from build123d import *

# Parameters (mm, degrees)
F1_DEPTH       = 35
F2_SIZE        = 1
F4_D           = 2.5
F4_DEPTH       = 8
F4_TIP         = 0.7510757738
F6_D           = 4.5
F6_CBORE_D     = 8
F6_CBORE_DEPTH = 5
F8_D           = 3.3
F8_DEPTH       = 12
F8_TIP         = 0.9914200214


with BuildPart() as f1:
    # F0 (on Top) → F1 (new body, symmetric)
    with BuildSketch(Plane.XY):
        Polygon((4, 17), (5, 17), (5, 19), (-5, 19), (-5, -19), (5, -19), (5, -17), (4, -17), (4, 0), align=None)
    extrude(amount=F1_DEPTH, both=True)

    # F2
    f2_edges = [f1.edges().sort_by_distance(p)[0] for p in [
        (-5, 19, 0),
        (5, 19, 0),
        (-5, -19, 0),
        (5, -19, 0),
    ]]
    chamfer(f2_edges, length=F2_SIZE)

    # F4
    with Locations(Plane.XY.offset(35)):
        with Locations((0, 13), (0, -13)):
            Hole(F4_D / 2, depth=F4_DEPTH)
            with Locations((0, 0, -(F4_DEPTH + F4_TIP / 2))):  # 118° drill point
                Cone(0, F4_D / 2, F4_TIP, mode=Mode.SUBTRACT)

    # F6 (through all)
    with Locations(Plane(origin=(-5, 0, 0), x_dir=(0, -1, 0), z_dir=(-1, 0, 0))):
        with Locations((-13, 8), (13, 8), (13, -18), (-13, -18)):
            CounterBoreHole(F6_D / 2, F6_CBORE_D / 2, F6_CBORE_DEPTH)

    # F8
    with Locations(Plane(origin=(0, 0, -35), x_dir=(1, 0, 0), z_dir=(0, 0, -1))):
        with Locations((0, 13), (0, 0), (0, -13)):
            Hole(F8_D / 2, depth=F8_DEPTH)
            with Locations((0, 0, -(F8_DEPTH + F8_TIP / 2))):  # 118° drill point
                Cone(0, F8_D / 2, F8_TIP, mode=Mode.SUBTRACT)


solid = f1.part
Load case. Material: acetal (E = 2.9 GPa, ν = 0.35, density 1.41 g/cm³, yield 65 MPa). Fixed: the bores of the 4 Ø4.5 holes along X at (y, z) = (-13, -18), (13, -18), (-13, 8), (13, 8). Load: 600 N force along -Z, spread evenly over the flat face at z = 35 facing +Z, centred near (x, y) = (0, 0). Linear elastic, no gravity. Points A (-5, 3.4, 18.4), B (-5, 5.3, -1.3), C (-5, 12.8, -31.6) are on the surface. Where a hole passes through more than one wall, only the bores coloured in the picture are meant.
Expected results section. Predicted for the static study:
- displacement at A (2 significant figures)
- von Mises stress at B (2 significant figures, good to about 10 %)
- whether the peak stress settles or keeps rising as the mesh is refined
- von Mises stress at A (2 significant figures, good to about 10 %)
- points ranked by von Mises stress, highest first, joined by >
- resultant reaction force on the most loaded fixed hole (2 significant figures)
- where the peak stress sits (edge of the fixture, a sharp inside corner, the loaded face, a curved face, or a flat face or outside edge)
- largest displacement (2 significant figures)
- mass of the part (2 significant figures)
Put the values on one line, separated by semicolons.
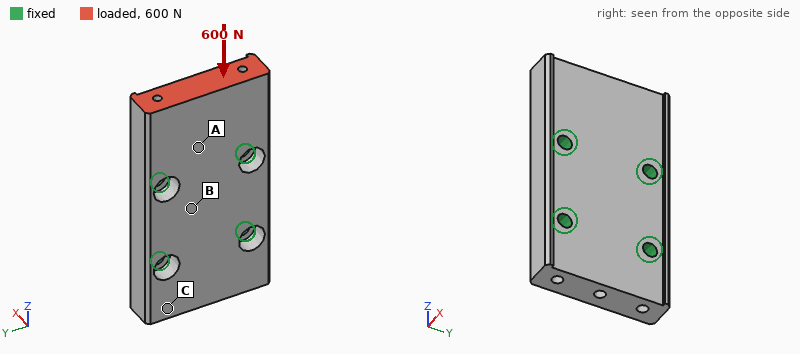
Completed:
28 µm; 1.5 MPa; keeps rising; 2.0 MPa; A > B > C; 220 N; edge of the fixture; 57 µm; 32 g
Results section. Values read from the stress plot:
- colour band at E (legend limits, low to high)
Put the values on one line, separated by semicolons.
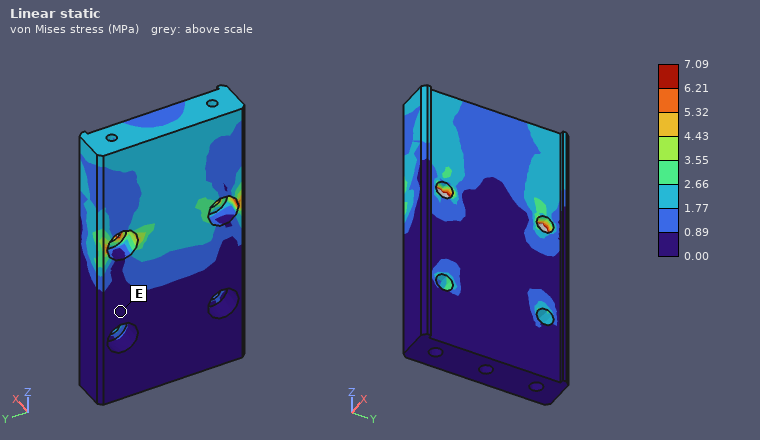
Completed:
0.00 to 0.89 MPa
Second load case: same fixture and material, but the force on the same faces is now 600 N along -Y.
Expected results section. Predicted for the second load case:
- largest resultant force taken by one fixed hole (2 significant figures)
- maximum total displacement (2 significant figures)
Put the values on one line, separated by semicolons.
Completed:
570 N; 0.15 mm
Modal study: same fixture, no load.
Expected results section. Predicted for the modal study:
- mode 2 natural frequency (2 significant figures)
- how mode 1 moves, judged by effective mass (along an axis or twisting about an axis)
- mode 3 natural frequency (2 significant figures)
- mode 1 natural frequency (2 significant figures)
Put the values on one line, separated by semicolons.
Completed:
3900 Hz; along X; 4000 Hz; 1900 Hz
